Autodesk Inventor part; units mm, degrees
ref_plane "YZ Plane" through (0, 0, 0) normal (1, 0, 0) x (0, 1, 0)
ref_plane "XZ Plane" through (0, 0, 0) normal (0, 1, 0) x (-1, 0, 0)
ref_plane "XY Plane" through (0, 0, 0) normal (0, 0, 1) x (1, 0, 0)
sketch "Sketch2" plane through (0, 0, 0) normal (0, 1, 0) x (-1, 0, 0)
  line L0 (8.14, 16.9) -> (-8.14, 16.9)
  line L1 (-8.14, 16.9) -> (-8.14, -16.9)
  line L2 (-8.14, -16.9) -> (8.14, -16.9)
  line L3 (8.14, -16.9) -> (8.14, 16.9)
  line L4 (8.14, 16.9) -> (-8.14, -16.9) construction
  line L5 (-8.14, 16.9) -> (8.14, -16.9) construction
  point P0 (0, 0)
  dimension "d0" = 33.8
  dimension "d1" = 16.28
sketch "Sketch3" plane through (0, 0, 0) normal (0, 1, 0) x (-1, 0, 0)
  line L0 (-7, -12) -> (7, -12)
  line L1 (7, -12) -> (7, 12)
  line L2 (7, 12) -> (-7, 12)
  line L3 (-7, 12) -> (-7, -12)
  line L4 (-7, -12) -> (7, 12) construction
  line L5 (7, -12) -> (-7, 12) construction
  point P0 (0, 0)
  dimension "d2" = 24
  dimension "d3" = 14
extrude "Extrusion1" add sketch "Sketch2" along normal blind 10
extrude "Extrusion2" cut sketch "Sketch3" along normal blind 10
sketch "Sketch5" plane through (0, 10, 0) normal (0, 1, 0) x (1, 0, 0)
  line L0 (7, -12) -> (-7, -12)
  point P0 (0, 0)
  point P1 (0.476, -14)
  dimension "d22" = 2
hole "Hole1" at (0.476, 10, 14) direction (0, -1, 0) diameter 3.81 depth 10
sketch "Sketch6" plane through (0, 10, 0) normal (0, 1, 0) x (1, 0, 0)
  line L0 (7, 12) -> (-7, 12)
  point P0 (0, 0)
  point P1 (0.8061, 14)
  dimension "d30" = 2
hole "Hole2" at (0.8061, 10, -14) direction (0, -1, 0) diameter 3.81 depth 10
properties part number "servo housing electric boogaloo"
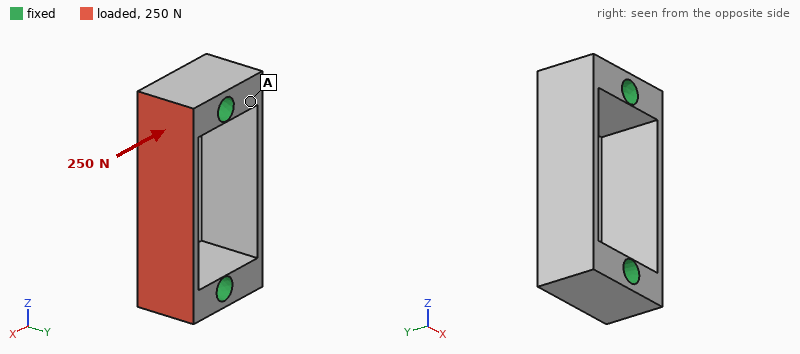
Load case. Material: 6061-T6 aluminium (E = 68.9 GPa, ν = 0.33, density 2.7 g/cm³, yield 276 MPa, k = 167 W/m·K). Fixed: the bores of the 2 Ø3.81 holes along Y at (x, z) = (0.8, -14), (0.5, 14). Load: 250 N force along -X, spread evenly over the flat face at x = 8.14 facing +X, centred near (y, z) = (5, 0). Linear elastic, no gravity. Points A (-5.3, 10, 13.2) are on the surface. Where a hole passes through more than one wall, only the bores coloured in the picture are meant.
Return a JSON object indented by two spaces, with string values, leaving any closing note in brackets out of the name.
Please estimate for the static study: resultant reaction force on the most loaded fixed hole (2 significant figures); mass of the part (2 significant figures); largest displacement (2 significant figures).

{
  "resultant reaction force on the most loaded fixed hole": "140 N",
  "mass of the part": "5.2 g",
  "largest displacement": "92 µm"
}
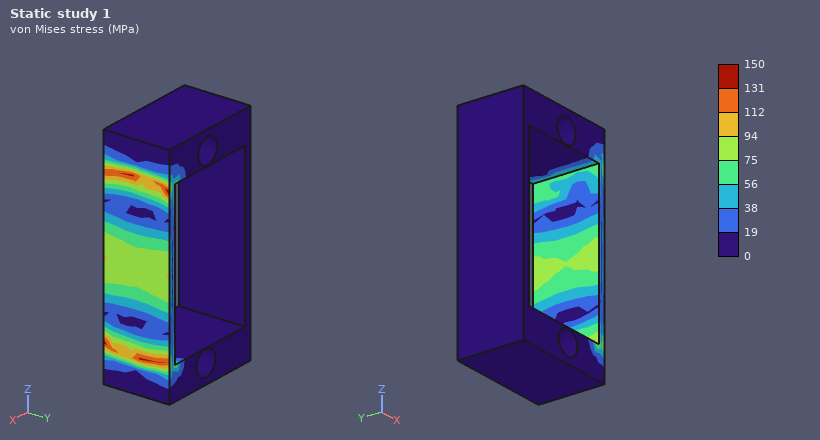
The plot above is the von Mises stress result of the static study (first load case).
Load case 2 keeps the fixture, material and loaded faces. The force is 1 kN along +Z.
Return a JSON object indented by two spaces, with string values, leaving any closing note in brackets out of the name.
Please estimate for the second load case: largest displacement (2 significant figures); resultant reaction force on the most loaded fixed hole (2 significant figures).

{
  "largest displacement": "12 µm",
  "resultant reaction force on the most loaded fixed hole": "520 N"
}
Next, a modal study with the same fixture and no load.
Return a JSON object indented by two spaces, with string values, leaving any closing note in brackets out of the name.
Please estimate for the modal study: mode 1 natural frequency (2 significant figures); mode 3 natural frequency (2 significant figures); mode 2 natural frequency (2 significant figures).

{
  "mode 1 natural frequency": "9500 Hz",
  "mode 3 natural frequency": "17 kHz",
  "mode 2 natural frequency": "9500 Hz"
}
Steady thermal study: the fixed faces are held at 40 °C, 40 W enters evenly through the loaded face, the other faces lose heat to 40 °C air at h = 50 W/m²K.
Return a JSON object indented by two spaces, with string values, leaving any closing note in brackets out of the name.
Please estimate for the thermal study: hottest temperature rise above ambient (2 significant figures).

{
  "hottest temperature rise above ambient": "63 K"
}
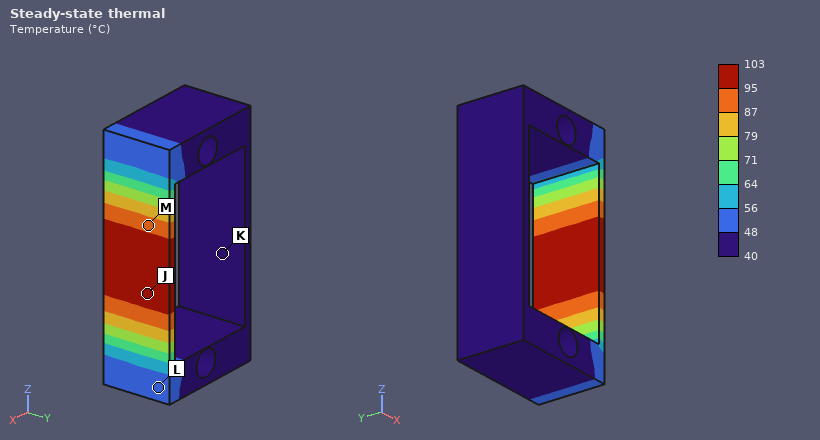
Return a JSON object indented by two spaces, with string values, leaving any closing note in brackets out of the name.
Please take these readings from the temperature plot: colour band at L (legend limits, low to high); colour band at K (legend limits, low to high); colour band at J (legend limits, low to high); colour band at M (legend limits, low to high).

{
  "colour band at L": "48 to 56 °C",
  "colour band at K": "40 to 48 °C",
  "colour band at J": "95 to 103 °C",
  "colour band at M": "87 to 95 °C"
}
